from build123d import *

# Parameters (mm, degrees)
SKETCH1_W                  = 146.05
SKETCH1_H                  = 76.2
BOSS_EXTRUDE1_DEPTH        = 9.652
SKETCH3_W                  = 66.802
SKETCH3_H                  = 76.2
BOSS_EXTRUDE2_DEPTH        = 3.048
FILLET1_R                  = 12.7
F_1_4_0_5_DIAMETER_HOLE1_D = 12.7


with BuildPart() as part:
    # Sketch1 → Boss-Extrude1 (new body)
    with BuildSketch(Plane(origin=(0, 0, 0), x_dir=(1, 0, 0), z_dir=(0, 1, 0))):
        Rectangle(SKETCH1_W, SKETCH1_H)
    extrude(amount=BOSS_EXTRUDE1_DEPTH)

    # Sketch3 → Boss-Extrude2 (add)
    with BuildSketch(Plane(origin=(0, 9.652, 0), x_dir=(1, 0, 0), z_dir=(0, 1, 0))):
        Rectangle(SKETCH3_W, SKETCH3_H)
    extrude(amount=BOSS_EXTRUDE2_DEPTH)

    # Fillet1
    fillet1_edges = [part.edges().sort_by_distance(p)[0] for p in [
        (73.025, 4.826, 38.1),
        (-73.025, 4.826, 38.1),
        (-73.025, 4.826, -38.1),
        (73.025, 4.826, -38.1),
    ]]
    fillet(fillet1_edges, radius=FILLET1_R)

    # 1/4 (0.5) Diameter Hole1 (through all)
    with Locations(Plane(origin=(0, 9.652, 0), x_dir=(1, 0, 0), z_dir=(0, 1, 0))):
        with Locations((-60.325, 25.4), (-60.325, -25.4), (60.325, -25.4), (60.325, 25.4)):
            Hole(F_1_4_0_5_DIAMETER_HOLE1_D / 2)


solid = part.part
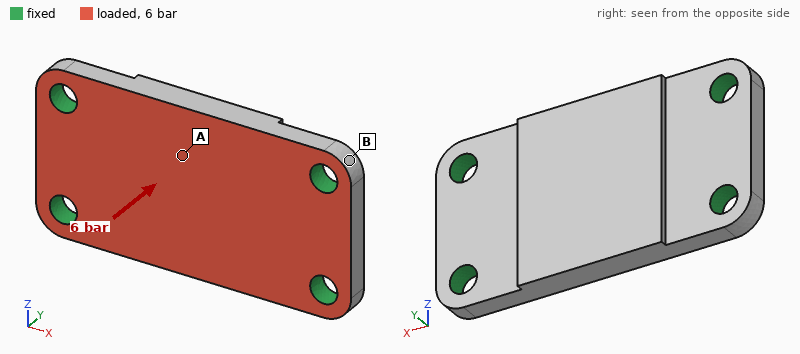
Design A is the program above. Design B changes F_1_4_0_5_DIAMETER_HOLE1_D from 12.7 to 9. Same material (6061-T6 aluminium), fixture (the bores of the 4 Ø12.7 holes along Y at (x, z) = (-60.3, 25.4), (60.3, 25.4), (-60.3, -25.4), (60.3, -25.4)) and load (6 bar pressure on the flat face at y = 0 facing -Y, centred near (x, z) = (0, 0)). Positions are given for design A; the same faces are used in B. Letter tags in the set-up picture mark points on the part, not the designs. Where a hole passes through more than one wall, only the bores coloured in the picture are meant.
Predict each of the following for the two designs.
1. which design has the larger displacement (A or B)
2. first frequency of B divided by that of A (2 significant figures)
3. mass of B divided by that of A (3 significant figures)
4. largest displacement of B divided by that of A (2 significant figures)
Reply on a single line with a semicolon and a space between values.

B; 0.92; 1.02; 1.2
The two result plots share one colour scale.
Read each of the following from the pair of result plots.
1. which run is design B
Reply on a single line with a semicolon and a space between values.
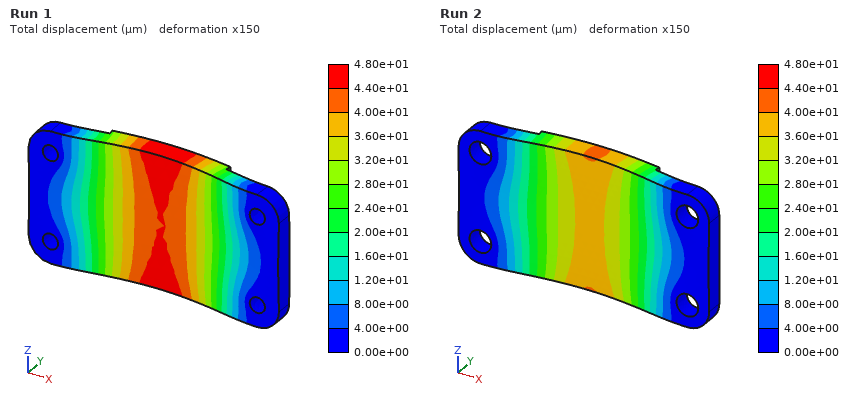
Run 1
